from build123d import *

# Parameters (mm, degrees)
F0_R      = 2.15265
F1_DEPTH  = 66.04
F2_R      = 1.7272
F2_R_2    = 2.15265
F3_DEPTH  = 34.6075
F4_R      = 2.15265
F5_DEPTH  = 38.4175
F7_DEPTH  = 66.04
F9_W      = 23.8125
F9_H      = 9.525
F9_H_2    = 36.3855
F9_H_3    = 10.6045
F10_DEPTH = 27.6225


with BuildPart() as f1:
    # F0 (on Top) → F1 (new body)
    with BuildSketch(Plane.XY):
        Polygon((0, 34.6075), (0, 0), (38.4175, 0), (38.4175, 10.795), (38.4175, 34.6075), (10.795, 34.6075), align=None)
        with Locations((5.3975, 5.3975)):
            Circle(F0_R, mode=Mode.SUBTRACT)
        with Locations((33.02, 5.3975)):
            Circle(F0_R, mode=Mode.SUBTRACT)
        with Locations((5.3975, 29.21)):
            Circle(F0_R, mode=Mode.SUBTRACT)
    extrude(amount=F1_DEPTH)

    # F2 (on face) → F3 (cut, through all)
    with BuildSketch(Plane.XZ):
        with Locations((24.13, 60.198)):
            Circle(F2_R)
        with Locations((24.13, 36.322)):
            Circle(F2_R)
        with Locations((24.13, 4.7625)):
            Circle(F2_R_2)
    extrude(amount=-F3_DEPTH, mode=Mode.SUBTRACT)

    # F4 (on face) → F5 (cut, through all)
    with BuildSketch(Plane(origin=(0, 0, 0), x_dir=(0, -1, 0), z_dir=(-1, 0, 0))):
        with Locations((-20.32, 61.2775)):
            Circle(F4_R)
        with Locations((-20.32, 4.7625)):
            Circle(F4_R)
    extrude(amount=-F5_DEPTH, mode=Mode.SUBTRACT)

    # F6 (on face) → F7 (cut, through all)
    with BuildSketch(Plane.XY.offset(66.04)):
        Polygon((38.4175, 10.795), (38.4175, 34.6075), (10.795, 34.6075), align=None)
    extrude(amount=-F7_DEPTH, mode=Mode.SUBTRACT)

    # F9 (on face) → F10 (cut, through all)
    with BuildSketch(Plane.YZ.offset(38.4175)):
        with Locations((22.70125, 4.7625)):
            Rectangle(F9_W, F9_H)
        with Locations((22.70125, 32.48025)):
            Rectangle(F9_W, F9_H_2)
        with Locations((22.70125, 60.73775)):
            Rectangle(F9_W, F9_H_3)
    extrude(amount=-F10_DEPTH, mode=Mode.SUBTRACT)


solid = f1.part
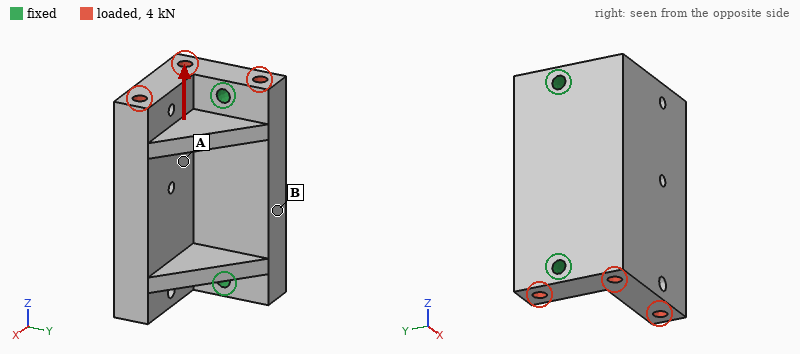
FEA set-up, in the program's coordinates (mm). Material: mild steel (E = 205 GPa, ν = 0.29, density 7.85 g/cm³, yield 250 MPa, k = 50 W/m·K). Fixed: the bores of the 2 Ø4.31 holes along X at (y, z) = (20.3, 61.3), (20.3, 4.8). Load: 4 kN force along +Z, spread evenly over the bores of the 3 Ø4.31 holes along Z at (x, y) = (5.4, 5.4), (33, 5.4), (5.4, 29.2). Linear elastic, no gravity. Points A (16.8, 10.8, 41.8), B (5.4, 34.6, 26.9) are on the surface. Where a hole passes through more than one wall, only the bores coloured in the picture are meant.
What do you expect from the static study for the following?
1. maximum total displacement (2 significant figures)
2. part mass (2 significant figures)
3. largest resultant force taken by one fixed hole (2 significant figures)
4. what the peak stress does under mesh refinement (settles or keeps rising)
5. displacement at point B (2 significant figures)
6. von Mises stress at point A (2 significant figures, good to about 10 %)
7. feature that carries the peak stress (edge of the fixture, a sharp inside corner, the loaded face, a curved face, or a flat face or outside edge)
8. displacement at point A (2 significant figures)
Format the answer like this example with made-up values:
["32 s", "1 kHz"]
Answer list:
["4.1 µm", "340 g", "2.2 kN", "keeps rising", "0.72 µm", "7.1 MPa", "edge of the fixture", "1.9 µm"]
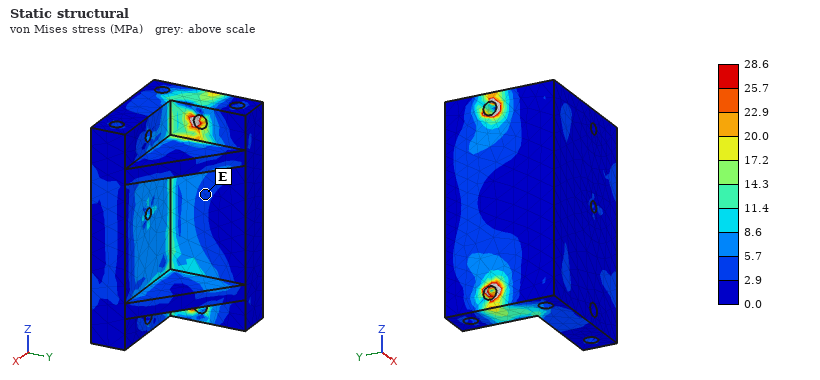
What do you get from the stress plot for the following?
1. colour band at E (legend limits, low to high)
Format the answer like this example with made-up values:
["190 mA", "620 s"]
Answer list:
["2.9 to 5.7 MPa"]
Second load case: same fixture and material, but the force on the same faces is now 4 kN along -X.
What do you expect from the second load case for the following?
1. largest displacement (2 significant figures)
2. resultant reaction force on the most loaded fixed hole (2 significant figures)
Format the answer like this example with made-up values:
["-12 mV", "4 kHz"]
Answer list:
["10 µm", "2.0 kN"]
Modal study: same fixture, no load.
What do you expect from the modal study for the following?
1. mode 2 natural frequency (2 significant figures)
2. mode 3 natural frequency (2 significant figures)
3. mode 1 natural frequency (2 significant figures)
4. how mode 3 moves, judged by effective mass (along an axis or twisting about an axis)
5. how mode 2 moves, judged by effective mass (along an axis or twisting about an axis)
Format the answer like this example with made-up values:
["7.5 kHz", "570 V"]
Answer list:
["8700 Hz", "12 kHz", "4800 Hz", "along X", "along Z"]
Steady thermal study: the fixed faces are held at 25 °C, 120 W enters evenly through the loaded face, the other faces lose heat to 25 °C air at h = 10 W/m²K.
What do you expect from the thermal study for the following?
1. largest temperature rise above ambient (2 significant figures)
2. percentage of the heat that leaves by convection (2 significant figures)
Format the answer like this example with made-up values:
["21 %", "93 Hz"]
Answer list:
["79 K", "5.4 %"]
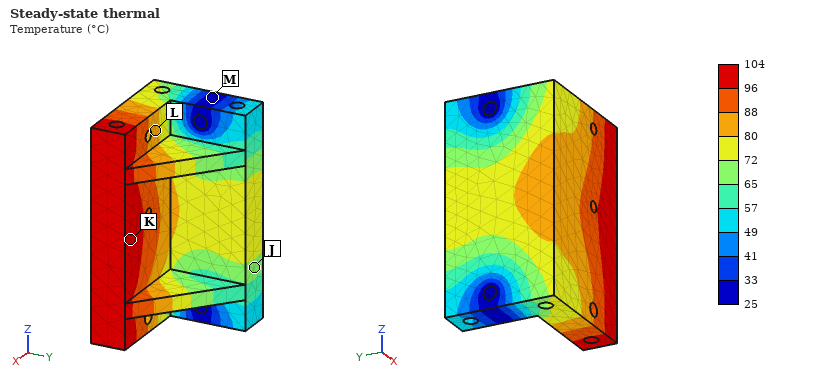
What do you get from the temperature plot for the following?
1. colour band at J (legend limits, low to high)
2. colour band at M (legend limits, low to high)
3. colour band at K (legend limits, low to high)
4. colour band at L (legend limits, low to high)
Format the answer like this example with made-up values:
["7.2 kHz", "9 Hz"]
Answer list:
["65 to 72 °C", "25 to 33 °C", "96 to 104 °C", "80 to 88 °C"]
